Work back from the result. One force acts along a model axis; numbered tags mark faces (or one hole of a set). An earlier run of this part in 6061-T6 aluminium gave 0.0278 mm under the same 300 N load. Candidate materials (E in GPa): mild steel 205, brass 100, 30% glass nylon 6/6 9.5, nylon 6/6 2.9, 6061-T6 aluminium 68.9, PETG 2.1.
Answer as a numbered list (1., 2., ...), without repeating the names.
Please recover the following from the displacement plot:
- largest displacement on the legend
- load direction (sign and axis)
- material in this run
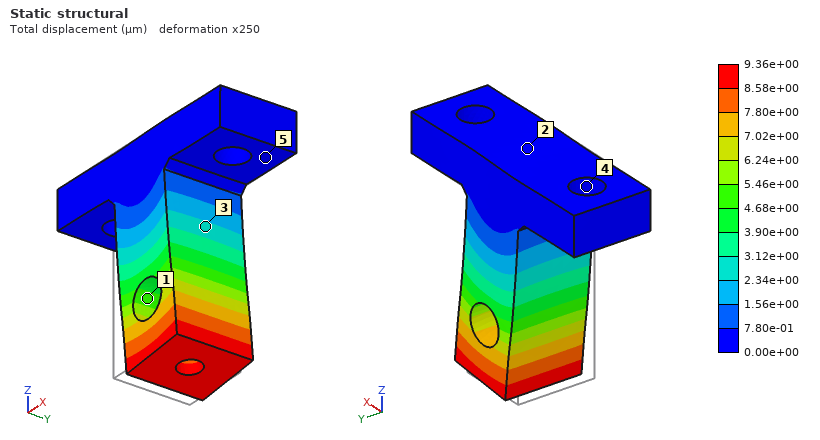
1. 9.36e+00 µm
2. +X
3. mild steel
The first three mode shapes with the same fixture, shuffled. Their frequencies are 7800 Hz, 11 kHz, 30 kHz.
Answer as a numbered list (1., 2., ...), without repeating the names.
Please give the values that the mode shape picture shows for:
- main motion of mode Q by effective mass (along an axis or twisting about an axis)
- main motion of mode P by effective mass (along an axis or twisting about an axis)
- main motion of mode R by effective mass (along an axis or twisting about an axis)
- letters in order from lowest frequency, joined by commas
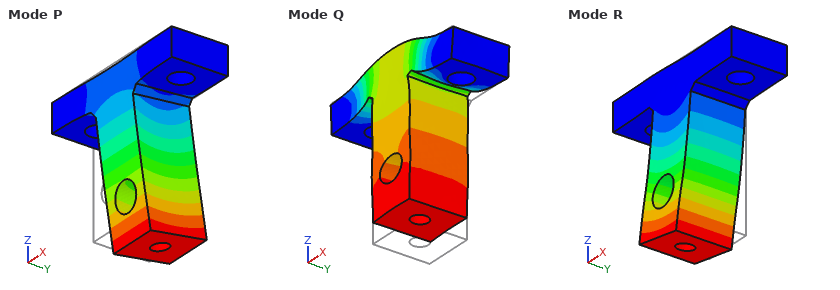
1. along Z
2. along Y
3. along X
4. P, R, Q
